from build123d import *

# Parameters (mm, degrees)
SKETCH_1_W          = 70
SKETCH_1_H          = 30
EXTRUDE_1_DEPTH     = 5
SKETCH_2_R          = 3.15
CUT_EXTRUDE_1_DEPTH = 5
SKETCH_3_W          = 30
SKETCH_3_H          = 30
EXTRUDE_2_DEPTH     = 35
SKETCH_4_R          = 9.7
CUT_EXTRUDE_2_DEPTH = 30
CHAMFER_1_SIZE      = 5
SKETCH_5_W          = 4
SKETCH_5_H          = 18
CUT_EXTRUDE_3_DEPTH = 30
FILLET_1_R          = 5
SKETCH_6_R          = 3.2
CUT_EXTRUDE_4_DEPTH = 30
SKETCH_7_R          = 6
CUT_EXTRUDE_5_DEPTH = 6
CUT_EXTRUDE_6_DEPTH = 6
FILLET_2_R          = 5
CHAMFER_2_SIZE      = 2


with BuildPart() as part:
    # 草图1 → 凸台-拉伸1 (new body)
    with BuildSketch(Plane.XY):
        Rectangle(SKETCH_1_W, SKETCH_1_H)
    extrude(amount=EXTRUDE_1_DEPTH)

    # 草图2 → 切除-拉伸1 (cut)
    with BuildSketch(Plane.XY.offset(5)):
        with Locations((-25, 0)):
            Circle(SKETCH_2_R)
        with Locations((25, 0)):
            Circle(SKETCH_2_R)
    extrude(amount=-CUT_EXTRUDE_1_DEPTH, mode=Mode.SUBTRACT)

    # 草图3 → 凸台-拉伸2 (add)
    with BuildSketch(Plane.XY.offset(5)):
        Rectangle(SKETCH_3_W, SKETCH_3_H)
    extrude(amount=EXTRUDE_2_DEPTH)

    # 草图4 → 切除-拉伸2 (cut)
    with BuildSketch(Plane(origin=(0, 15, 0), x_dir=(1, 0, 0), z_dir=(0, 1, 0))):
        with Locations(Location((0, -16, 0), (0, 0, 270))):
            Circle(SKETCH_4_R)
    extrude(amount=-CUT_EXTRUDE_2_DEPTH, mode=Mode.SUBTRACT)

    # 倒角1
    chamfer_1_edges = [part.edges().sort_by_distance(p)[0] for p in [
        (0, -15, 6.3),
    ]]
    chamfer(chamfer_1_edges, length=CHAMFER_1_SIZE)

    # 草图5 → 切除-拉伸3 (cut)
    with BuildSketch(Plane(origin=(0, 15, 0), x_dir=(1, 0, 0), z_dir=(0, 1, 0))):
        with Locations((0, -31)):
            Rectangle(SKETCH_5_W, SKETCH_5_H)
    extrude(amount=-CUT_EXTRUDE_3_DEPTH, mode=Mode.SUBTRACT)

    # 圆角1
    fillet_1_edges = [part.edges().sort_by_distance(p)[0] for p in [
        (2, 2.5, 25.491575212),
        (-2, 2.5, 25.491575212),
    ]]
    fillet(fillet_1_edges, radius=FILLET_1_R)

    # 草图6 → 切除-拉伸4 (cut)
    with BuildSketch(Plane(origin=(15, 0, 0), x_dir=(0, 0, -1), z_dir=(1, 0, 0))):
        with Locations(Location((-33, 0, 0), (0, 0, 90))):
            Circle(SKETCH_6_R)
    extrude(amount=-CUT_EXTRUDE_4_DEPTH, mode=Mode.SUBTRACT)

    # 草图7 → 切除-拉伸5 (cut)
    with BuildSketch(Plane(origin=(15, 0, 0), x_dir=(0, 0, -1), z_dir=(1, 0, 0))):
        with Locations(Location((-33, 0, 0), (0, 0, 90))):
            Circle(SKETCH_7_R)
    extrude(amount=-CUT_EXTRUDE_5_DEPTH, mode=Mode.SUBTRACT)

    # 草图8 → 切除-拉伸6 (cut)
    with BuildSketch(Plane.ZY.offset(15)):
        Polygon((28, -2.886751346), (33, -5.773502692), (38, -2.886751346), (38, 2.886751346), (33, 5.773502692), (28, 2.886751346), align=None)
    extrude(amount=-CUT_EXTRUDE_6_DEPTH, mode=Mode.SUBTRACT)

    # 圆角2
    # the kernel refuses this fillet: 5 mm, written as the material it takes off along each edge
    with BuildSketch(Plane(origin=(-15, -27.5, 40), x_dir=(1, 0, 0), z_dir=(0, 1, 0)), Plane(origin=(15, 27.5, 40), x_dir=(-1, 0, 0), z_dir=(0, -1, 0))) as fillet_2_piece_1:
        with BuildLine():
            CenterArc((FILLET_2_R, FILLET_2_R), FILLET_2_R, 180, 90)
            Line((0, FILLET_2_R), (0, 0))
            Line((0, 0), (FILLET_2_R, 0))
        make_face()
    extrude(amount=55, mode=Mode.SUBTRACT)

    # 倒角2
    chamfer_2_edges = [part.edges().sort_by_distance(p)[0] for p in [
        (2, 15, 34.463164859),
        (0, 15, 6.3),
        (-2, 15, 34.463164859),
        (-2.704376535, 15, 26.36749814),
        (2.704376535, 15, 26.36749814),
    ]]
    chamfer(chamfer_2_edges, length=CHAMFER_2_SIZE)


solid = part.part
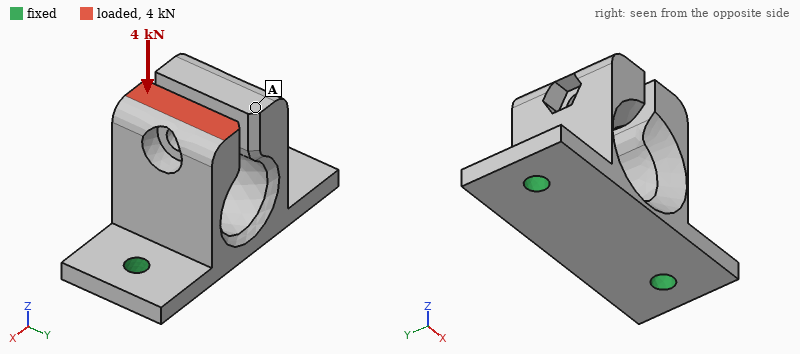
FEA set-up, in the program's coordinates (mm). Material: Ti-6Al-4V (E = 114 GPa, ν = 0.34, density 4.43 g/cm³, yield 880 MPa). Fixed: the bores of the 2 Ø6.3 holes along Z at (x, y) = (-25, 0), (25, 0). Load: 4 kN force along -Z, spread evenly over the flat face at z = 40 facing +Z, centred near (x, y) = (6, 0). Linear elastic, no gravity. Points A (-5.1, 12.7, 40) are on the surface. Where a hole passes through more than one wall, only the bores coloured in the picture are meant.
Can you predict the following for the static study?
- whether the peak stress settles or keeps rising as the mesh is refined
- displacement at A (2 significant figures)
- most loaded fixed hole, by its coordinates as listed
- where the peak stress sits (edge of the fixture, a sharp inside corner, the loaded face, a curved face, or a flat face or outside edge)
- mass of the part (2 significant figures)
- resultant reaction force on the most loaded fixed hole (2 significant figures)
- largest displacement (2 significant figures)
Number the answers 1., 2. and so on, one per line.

1. keeps rising
2. 0.074 mm
3. (25, 0)
4. edge of the fixture
5. 120 g
6. 2.9 kN
7. 0.27 mm
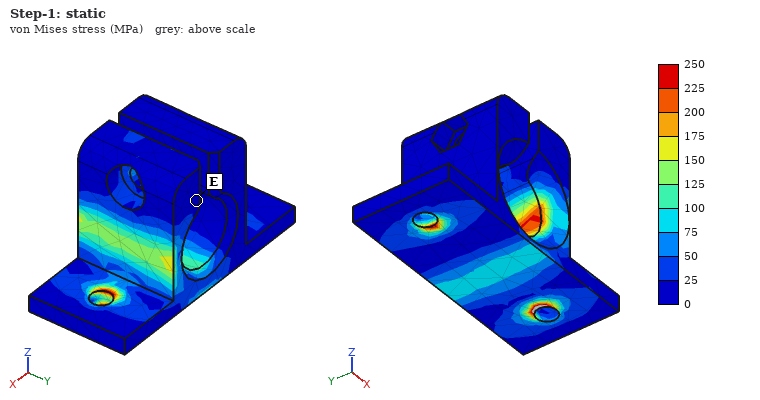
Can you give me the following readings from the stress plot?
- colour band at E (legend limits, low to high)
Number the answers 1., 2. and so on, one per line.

1. 0 to 25 MPa
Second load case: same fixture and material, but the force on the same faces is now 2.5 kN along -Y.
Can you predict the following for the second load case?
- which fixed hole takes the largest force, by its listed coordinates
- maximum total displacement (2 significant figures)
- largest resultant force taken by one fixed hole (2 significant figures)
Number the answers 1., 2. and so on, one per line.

1. (25, 0)
2. 0.42 mm
3. 1.5 kN
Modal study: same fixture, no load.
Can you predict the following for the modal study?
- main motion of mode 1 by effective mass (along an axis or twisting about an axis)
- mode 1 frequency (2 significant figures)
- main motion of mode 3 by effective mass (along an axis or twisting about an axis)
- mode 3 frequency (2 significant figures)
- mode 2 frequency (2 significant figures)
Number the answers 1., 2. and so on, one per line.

1. along Y
2. 2400 Hz
3. along X
4. 3000 Hz
5. 2500 Hz
